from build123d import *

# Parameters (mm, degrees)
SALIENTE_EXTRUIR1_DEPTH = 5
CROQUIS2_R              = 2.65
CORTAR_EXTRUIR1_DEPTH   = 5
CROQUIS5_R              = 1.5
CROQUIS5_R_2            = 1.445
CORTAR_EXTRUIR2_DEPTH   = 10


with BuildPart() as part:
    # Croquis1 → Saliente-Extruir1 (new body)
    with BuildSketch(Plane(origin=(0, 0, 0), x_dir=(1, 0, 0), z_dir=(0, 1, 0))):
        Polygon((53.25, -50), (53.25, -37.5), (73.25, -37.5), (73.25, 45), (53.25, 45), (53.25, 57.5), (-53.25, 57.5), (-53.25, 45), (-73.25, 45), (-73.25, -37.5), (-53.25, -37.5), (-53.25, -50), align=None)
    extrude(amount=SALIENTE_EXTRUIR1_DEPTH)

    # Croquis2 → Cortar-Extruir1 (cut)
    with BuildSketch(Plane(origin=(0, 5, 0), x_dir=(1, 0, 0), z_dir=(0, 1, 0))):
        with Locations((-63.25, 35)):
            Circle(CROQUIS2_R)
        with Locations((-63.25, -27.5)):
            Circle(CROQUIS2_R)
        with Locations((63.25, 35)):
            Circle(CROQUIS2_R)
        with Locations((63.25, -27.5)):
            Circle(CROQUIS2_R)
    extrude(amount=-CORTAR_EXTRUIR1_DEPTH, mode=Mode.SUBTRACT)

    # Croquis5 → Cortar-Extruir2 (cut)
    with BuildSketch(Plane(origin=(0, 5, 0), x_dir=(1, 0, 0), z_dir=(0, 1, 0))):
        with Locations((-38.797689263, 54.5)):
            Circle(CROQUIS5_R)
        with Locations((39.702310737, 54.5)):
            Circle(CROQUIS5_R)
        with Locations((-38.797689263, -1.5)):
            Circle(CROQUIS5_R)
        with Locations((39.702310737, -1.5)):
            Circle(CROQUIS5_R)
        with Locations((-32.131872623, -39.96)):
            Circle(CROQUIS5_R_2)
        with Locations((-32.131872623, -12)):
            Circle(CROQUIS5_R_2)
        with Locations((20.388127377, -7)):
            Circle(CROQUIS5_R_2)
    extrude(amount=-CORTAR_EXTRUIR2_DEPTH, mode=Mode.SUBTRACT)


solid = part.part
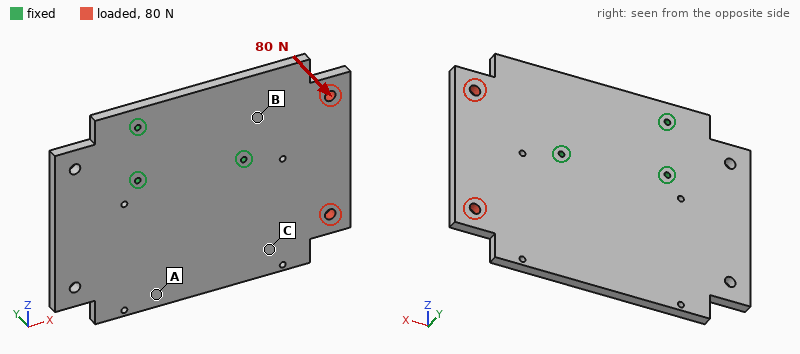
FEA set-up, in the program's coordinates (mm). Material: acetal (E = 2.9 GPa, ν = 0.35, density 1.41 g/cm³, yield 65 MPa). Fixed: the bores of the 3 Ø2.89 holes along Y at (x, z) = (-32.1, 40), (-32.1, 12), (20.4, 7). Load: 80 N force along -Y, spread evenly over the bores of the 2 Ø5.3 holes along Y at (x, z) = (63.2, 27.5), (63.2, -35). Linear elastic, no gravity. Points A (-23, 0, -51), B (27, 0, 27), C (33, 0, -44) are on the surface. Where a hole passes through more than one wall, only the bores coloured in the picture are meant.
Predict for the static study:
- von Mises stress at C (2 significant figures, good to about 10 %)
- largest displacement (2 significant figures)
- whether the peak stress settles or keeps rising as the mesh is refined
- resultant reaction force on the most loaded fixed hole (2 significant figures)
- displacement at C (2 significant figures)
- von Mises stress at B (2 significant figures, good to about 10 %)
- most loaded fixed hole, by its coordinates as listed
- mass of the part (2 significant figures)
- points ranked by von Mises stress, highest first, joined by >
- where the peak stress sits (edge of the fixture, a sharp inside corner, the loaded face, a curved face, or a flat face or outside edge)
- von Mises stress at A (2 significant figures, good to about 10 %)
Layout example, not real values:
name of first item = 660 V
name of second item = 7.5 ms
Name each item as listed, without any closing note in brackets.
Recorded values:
von Mises stress at C = 3.5 MPa
largest displacement = 2.1 mm
whether the peak stress settles or keeps rising as the mesh is refined = keeps rising
resultant reaction force on the most loaded fixed hole = 130 N
displacement at C = 0.76 mm
von Mises stress at B = 5.6 MPa
most loaded fixed hole, by its coordinates as listed = (20.4, 7)
mass of the part = 100 g
points ranked by von Mises stress, highest first, joined by > = B > C > A
where the peak stress sits = edge of the fixture
von Mises stress at A = 1.7 MPa
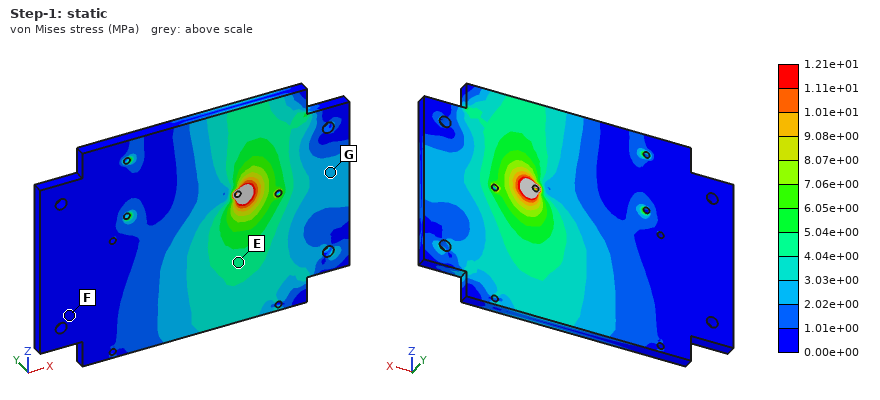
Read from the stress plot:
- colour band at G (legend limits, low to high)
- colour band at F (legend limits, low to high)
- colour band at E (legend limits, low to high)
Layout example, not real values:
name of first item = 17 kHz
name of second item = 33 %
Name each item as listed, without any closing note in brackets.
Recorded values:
colour band at G = 2.02e+00 to 3.03e+00 MPa
colour band at F = 0.00e+00 to 1.01e+00 MPa
colour band at E = 4.04e+00 to 5.04e+00 MPa
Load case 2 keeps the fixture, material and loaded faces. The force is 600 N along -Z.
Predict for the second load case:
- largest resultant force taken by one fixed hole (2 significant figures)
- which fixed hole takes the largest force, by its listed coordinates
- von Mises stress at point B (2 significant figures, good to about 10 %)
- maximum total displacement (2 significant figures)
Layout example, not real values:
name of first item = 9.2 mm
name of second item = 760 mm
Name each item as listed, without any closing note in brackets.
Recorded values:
largest resultant force taken by one fixed hole = 910 N
which fixed hole takes the largest force, by its listed coordinates = (20.4, 7)
von Mises stress at point B = 3.1 MPa
maximum total displacement = 0.25 mm
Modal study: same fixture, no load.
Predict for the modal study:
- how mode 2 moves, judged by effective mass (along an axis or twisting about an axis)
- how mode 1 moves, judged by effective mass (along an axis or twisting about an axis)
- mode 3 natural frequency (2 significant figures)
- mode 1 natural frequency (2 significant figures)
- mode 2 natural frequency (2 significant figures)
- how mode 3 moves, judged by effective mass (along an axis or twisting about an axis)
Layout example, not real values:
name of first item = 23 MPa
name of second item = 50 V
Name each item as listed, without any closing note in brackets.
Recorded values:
how mode 2 moves, judged by effective mass = twisting about Z
how mode 1 moves, judged by effective mass = along Y
mode 3 natural frequency = 390 Hz
mode 1 natural frequency = 220 Hz
mode 2 natural frequency = 290 Hz
how mode 3 moves, judged by effective mass = along Y
